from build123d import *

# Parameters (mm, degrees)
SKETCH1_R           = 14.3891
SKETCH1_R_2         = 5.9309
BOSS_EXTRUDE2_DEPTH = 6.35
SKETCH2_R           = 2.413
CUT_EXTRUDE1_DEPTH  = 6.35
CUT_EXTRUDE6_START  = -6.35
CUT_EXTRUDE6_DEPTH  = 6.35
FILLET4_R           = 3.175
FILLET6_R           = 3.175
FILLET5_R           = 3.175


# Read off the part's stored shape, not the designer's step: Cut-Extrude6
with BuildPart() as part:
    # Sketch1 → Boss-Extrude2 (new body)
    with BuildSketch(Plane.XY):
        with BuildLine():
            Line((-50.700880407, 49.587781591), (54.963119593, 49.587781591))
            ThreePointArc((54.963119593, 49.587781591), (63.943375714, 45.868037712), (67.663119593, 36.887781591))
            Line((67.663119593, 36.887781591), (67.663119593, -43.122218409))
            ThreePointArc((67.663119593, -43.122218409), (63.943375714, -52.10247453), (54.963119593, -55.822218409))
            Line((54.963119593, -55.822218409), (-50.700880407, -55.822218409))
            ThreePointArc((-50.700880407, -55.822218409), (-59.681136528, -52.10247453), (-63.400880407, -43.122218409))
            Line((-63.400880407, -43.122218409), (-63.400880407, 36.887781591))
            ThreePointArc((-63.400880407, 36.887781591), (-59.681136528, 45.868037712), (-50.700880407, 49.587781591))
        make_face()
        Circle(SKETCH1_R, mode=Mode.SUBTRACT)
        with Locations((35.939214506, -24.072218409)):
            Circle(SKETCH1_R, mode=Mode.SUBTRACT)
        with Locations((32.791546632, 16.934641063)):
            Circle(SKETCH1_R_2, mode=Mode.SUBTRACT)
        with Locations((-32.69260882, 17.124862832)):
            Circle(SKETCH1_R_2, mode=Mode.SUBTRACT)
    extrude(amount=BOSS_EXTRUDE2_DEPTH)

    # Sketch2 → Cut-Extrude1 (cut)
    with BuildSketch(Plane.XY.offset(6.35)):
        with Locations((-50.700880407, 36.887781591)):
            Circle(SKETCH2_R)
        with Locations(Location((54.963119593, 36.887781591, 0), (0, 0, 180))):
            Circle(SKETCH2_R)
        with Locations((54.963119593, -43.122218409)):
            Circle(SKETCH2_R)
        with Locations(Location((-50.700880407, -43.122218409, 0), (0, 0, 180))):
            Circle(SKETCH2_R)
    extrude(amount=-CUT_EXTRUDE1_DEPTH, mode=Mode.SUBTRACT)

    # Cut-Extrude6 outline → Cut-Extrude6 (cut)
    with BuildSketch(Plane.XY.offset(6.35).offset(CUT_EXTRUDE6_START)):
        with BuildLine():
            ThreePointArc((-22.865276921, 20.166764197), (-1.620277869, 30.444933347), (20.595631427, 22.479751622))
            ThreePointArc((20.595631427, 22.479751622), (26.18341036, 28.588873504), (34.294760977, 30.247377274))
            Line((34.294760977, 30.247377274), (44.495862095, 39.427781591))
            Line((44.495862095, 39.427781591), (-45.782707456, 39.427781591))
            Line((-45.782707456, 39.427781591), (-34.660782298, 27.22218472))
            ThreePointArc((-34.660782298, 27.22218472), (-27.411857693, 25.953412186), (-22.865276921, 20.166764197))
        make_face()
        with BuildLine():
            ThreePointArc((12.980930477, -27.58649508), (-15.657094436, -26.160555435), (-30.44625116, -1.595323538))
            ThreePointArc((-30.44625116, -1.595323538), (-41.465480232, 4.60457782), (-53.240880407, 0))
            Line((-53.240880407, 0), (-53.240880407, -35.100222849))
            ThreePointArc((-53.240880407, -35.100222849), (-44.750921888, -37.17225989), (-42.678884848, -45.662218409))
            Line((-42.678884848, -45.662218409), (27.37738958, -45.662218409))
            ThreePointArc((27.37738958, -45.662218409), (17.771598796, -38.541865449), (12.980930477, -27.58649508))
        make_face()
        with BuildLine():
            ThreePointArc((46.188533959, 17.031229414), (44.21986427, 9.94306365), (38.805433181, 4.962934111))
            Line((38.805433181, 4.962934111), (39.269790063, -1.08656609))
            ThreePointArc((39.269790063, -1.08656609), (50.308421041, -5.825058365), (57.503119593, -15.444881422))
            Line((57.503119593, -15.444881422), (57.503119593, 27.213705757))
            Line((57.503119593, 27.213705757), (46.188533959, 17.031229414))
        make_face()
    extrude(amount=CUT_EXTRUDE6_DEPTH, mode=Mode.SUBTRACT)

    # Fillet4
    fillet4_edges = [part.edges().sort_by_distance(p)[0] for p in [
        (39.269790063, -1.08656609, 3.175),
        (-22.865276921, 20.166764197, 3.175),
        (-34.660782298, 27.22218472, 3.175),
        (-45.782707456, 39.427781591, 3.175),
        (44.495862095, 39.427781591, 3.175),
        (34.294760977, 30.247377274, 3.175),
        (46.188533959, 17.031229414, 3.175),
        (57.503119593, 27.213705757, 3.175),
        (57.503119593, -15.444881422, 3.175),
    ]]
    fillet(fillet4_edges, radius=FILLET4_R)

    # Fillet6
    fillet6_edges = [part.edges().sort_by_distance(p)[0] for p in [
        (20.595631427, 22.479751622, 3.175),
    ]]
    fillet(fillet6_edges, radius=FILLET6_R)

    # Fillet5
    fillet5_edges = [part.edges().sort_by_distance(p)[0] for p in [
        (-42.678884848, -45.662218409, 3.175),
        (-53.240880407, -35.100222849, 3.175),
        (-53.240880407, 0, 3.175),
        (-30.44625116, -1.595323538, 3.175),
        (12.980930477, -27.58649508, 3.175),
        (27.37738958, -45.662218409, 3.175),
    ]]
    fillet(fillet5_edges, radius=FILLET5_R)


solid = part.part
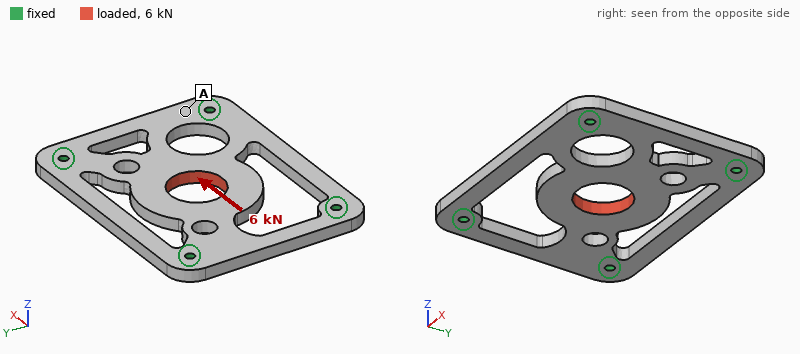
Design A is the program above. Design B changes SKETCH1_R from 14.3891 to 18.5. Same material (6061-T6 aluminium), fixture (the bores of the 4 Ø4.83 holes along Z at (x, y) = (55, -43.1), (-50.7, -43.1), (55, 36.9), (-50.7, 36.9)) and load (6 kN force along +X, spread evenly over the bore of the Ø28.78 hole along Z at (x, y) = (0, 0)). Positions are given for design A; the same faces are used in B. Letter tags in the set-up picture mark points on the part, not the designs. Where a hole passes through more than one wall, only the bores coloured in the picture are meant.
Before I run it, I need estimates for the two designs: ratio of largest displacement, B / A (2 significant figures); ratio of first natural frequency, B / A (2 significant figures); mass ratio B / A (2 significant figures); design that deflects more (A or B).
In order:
1.7
1.0
0.90
B
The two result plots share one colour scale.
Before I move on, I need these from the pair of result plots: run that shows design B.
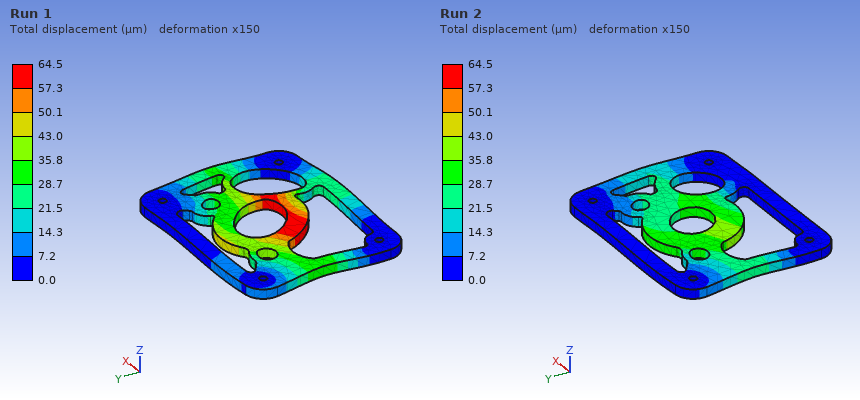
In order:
Run 1
